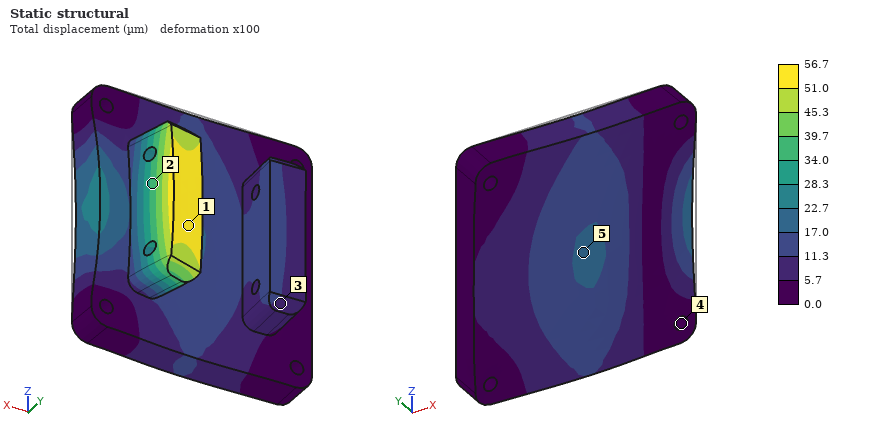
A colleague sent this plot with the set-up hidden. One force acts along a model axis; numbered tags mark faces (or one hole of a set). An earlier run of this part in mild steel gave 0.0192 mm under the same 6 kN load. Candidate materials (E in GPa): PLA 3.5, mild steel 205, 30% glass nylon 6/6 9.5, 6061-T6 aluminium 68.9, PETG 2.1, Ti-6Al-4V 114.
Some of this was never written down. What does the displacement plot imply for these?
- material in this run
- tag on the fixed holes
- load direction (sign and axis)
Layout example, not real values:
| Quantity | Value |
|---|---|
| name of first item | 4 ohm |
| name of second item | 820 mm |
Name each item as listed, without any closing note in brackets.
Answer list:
| Quantity | Value |
|---|---|
| material in this run | 6061-T6 aluminium |
| tag on the fixed holes | 4 |
| load direction | -X |
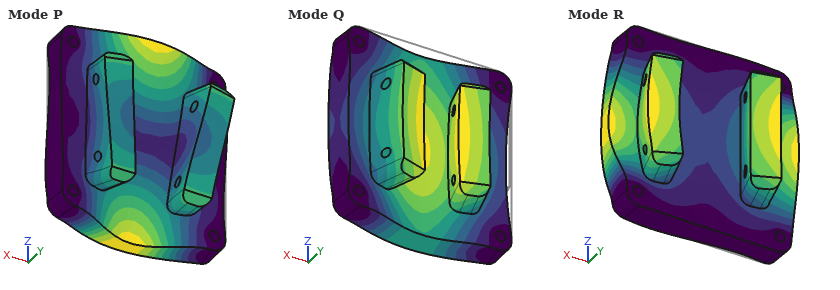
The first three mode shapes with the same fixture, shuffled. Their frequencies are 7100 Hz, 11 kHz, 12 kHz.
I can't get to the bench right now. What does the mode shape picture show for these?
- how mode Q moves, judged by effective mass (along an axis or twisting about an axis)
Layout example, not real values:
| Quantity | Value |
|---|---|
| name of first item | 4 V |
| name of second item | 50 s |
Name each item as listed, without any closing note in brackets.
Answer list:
| Quantity | Value |
|---|---|
| how mode Q moves, judged by effective mass | along Y |
